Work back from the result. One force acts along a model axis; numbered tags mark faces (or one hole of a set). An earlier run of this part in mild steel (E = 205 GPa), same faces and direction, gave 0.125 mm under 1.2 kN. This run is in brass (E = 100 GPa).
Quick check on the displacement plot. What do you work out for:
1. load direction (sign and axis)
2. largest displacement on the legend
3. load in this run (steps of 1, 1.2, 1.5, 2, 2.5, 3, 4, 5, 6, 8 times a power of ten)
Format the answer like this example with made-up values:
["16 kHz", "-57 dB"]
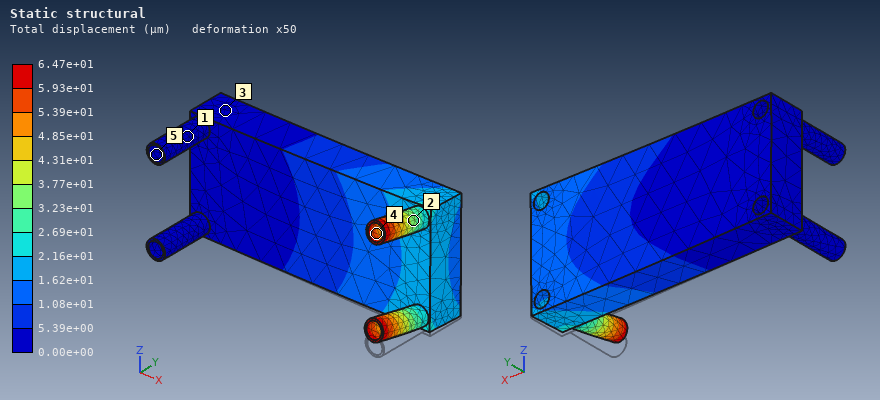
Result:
["+Z", "6.47e+01 µm", "300 N"]
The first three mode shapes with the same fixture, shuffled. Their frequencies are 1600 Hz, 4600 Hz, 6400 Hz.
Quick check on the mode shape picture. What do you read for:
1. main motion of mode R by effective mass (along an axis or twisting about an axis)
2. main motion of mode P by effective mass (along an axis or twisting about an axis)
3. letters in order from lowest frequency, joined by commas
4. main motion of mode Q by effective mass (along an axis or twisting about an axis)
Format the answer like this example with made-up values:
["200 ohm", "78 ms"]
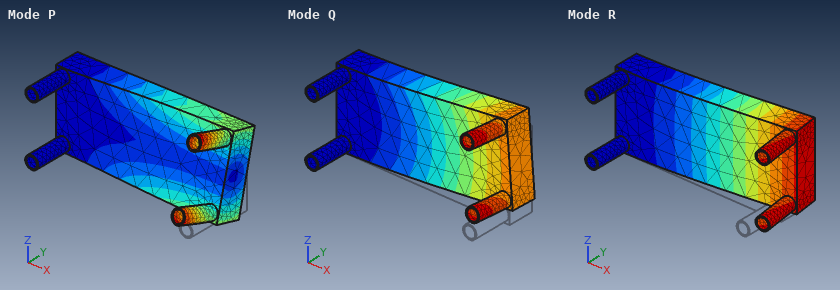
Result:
["along Y", "twisting about X", "R, Q, P", "along Z"]
